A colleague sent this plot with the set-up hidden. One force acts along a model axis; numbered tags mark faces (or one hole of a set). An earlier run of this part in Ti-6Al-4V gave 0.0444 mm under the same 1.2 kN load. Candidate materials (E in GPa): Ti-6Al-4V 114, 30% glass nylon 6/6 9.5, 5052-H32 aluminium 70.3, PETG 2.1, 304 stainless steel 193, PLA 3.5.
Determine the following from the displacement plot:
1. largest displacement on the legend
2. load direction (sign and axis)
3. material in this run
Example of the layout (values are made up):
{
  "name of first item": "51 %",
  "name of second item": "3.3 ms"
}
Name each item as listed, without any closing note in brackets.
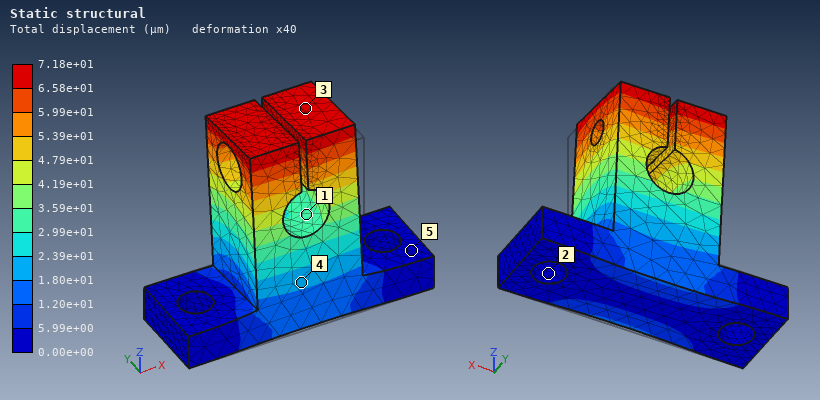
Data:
{
  "largest displacement on the legend": "7.18e+01 µm",
  "load direction": "+Y",
  "material in this run": "5052-H32 aluminium"
}
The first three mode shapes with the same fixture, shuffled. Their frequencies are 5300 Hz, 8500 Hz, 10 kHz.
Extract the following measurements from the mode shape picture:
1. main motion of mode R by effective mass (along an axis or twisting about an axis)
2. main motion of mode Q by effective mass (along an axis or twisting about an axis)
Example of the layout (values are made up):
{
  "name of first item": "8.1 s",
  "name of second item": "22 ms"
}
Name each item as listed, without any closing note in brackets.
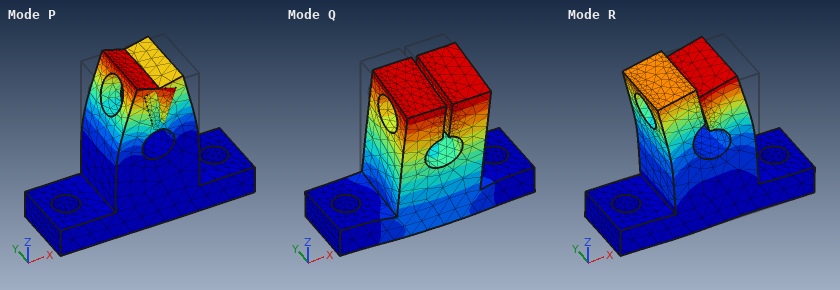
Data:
{
  "main motion of mode R by effective mass": "along X",
  "main motion of mode Q by effective mass": "along Y"
}
